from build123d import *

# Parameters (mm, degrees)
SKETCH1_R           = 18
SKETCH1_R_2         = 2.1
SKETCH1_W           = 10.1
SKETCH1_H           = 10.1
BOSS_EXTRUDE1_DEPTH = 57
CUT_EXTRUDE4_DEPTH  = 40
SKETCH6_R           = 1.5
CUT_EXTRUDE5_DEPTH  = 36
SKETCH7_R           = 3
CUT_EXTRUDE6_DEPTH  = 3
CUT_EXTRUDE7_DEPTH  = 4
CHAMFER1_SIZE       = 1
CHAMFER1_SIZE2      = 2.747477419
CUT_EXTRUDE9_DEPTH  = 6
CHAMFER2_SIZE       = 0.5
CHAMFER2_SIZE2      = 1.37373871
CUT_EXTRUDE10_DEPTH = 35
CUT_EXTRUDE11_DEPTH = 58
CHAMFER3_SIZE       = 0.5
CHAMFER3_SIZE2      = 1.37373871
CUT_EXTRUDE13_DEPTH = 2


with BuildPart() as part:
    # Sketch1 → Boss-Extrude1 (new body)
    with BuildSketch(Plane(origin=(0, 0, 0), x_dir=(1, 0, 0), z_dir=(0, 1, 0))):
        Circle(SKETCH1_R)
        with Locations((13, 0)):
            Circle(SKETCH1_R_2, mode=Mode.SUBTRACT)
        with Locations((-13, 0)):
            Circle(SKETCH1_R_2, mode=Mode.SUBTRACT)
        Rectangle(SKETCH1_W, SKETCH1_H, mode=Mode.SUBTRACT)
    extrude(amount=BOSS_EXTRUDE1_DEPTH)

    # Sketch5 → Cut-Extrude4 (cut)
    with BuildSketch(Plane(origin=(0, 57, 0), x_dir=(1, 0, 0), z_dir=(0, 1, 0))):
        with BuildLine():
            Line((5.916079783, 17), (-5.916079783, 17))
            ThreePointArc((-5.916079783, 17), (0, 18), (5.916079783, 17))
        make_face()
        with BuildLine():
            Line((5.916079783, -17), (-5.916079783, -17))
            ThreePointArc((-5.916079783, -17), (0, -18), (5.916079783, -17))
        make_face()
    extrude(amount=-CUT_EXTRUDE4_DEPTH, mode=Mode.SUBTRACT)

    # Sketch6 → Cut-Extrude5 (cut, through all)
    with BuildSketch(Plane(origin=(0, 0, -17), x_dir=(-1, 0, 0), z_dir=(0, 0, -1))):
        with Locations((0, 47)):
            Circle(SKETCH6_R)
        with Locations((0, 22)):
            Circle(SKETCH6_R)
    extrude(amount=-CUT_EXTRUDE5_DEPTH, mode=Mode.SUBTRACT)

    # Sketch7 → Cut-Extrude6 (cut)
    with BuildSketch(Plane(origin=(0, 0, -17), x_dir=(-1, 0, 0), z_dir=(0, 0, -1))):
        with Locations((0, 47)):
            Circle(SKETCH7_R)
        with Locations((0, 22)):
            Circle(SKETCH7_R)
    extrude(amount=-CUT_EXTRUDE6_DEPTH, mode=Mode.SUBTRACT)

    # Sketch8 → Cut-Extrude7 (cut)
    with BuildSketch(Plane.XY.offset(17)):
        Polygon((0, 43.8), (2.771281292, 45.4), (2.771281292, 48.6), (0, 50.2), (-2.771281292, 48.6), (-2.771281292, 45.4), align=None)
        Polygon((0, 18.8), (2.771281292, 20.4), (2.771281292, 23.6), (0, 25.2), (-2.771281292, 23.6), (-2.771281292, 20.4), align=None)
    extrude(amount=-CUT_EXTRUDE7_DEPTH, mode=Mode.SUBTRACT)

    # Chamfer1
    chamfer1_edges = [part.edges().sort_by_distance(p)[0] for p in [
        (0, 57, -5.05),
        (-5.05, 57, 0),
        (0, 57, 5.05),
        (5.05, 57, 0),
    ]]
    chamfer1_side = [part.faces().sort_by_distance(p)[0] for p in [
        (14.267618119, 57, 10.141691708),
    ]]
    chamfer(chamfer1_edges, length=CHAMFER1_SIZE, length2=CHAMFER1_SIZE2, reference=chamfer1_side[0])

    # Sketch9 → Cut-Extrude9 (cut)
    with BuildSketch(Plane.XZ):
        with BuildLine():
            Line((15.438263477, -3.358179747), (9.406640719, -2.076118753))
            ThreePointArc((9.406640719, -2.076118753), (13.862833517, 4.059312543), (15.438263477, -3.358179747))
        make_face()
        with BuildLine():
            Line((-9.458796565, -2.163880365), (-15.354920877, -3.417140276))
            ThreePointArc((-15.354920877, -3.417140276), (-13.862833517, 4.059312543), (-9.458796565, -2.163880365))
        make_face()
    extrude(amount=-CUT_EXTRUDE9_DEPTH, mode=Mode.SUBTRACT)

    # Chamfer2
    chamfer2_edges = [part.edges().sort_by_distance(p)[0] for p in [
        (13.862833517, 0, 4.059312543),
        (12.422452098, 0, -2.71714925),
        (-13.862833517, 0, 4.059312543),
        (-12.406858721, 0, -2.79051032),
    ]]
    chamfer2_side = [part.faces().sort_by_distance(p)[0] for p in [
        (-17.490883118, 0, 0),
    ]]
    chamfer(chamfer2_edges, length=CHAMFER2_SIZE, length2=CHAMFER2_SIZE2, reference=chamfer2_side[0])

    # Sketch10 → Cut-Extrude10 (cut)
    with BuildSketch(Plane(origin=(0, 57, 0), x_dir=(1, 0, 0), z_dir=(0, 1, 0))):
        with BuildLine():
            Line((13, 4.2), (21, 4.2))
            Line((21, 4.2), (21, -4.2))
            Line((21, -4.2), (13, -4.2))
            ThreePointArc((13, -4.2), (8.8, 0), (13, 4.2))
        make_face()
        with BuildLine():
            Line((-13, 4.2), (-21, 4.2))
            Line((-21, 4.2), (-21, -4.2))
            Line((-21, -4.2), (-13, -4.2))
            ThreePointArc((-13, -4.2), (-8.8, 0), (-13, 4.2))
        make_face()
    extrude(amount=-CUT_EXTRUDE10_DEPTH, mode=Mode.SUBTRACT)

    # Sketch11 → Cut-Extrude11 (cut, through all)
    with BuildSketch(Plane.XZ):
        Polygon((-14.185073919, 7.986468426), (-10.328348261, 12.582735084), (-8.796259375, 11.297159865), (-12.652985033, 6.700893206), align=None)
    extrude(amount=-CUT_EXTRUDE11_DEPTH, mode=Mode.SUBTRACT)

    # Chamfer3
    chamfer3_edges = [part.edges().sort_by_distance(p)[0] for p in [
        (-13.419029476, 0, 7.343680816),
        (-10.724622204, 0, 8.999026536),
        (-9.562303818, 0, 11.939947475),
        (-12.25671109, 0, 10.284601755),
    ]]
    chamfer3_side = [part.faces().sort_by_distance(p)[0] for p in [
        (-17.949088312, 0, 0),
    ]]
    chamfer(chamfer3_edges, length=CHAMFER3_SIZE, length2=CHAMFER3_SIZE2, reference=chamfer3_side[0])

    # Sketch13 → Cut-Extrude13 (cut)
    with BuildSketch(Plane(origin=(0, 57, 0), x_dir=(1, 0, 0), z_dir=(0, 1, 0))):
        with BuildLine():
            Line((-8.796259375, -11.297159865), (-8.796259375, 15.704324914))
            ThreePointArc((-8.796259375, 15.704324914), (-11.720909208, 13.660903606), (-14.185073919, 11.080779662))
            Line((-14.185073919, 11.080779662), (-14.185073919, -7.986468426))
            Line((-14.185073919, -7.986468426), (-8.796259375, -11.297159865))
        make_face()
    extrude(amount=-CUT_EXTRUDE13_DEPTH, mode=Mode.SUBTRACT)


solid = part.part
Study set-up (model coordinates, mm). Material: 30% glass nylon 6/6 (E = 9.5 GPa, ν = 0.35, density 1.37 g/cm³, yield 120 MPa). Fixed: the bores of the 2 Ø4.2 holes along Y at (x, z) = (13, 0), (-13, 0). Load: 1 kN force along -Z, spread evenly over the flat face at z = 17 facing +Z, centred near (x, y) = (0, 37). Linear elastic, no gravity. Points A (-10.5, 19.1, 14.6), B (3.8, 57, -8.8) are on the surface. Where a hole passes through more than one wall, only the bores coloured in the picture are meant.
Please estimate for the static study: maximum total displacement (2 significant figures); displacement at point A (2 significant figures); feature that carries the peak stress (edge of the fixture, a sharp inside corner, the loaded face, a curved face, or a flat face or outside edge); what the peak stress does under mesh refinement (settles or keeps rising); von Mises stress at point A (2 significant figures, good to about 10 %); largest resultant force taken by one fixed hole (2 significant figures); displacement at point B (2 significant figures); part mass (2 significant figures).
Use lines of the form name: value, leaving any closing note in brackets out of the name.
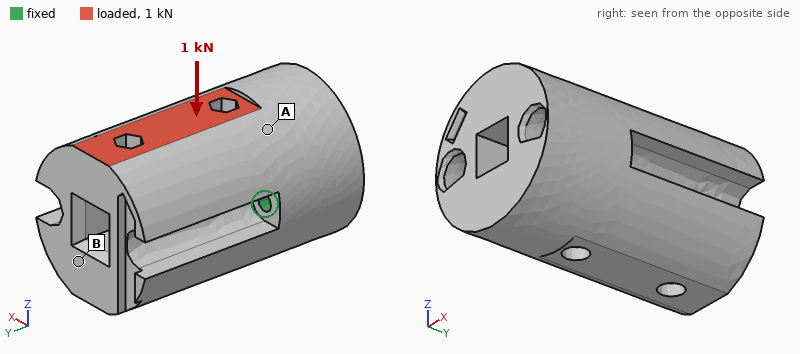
maximum total displacement: 100 µm
displacement at point A: 24 µm
feature that carries the peak stress: edge of the fixture
what the peak stress does under mesh refinement: keeps rising
von Mises stress at point A: 5.2 MPa
largest resultant force taken by one fixed hole: 500 N
displacement at point B: 88 µm
part mass: 61 g
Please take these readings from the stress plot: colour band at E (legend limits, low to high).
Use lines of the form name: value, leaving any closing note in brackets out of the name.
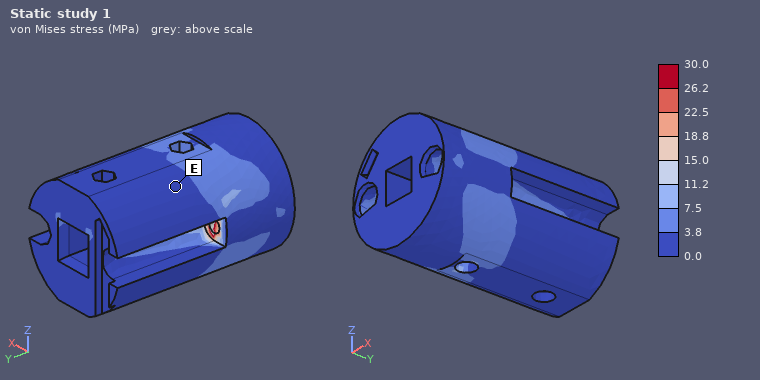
colour band at E: 0.0 to 3.8 MPa
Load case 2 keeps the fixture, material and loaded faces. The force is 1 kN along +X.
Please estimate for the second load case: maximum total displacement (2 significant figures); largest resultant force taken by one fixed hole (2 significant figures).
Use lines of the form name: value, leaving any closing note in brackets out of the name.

maximum total displacement: 63 µm
largest resultant force taken by one fixed hole: 1.1 kN
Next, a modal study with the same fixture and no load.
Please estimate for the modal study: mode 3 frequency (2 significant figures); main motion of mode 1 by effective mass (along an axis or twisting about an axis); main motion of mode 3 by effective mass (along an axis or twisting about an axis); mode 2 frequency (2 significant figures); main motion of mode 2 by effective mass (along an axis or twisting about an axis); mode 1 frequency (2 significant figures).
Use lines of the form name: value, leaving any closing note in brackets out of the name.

mode 3 frequency: 7800 Hz
main motion of mode 1 by effective mass: along Z
main motion of mode 3 by effective mass: twisting about Y
mode 2 frequency: 4900 Hz
main motion of mode 2 by effective mass: along X
mode 1 frequency: 3100 Hz
